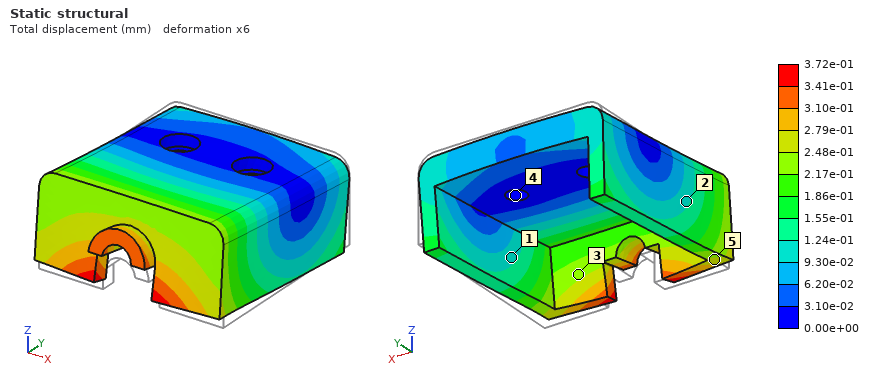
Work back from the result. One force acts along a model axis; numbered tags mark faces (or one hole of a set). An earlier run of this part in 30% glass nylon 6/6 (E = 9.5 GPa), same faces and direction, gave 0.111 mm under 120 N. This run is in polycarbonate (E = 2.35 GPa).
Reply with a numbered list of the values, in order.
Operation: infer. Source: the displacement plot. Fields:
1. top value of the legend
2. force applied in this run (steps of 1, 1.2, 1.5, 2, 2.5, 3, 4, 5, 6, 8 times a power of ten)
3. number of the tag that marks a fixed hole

1. 3.72e-01 mm
2. 100 N
3. 4
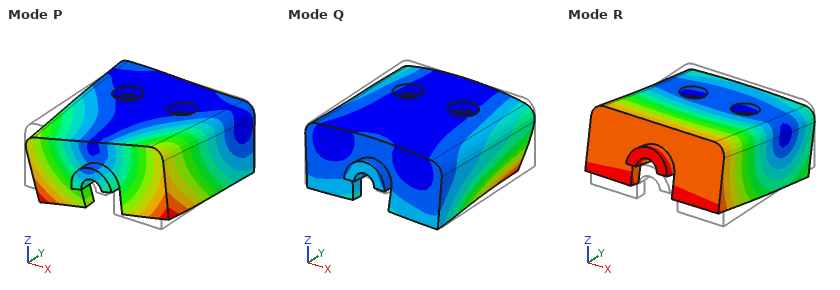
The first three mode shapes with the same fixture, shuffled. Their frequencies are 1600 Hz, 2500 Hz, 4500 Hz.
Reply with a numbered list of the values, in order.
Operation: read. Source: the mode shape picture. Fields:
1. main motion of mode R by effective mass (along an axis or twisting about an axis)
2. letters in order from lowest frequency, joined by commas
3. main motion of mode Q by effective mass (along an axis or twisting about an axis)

1. along Z
2. R, P, Q
3. along Z
